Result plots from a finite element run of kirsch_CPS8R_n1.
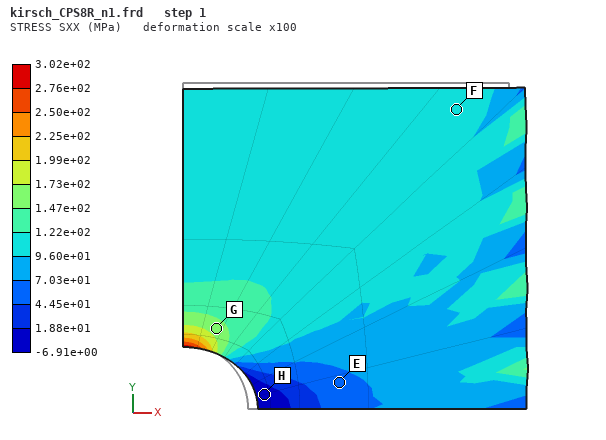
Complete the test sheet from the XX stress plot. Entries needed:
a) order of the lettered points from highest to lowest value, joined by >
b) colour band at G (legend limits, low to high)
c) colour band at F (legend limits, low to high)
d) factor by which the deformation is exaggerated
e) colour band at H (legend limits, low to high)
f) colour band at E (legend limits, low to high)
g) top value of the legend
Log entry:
G > F > E > H
1.47e+02 to 1.73e+02 MPa
9.60e+01 to 1.22e+02 MPa
100
-6.91e+00 to 1.88e+01 MPa
4.45e+01 to 7.03e+01 MPa
3.02e+02 MPa
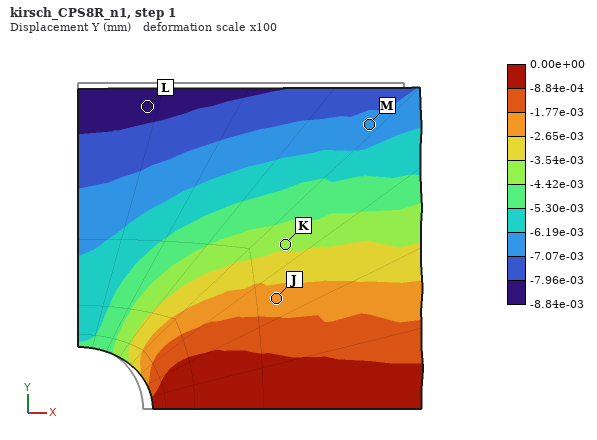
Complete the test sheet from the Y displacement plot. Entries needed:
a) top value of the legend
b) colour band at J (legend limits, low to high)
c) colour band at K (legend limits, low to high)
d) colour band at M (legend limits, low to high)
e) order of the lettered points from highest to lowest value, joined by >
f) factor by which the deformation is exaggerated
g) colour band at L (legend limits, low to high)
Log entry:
0.00e+00 mm
-2.65e-03 to -1.77e-03 mm
-4.42e-03 to -3.54e-03 mm
-7.07e-03 to -6.19e-03 mm
J > K > M > L
100
-8.84e-03 to -7.96e-03 mm
